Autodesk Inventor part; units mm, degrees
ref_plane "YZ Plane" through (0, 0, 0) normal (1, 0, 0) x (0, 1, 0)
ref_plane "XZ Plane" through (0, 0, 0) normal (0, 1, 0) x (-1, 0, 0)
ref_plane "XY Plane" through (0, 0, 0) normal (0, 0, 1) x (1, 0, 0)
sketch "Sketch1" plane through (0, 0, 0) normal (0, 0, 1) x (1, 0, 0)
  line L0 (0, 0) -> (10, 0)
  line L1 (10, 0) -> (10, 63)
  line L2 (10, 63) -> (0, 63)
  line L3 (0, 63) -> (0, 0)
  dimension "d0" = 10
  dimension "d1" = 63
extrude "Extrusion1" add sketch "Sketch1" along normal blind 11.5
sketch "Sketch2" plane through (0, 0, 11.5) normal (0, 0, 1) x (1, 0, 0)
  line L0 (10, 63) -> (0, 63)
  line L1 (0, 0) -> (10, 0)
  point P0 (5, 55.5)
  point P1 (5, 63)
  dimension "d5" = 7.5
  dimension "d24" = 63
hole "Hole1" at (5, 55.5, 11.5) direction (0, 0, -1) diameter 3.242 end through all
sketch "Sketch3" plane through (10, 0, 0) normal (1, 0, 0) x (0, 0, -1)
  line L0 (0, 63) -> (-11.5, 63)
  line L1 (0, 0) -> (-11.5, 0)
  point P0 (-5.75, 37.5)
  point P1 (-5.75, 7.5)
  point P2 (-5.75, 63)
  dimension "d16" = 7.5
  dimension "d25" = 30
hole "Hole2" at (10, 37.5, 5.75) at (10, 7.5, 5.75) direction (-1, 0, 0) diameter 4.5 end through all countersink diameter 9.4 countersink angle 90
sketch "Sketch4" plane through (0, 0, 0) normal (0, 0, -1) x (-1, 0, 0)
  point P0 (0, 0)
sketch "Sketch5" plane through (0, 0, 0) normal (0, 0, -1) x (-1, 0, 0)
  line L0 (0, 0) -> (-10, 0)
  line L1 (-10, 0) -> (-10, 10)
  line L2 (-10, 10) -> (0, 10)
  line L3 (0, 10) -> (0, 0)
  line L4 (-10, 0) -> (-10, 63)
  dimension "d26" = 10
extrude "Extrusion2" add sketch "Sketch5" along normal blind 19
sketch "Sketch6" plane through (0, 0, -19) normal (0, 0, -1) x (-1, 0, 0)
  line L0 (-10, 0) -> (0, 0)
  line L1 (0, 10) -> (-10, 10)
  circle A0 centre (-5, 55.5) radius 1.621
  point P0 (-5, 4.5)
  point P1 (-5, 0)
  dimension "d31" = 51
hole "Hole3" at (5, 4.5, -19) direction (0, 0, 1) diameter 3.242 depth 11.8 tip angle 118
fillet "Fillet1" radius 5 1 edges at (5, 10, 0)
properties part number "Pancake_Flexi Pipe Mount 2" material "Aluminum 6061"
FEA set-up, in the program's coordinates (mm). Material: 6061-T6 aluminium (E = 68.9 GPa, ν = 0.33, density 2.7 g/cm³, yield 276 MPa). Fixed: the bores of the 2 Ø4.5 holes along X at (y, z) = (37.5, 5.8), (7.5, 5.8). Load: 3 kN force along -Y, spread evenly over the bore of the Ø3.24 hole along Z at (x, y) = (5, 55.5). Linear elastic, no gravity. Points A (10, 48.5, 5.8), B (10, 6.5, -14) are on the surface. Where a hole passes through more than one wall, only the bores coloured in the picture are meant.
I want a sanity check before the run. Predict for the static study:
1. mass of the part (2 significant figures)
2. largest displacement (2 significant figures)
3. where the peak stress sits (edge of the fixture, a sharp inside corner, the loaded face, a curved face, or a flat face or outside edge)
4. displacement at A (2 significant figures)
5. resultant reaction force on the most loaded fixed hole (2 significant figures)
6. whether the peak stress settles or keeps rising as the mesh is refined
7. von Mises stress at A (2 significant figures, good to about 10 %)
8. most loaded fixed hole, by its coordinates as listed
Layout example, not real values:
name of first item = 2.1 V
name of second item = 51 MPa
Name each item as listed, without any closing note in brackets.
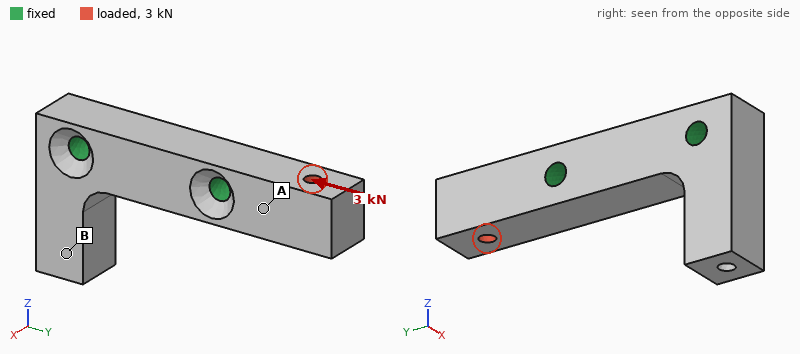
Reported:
mass of the part = 23 g
largest displacement = 10 µm
where the peak stress sits = edge of the fixture
displacement at A = 6.6 µm
resultant reaction force on the most loaded fixed hole = 2.9 kN
whether the peak stress settles or keeps rising as the mesh is refined = keeps rising
von Mises stress at A = 26 MPa
most loaded fixed hole, by its coordinates as listed = (37.5, 5.8)
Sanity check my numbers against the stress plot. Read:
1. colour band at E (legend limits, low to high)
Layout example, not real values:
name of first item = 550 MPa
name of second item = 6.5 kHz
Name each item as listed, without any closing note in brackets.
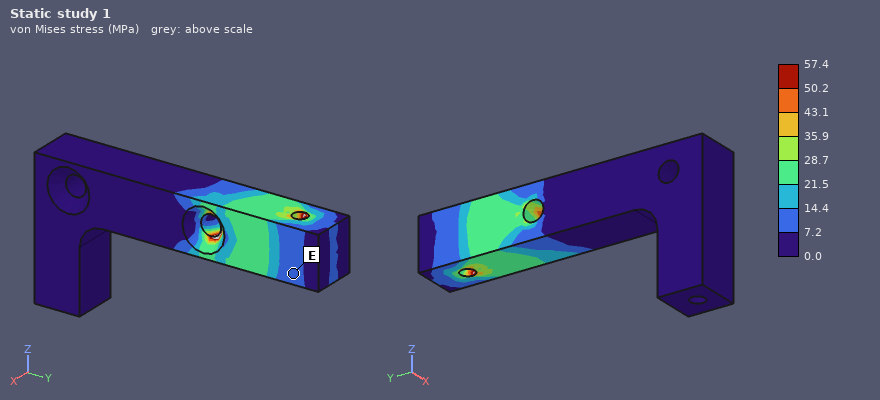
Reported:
colour band at E = 7.2 to 14.4 MPa
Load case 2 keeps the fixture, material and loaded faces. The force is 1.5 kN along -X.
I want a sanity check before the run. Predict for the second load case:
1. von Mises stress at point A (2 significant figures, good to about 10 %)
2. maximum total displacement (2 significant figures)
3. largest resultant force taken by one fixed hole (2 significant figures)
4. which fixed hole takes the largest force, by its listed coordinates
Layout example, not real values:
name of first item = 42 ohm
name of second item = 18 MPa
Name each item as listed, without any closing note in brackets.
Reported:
von Mises stress at point A = 53 MPa
maximum total displacement = 0.10 mm
largest resultant force taken by one fixed hole = 1.7 kN
which fixed hole takes the largest force, by its listed coordinates = (37.5, 5.8)
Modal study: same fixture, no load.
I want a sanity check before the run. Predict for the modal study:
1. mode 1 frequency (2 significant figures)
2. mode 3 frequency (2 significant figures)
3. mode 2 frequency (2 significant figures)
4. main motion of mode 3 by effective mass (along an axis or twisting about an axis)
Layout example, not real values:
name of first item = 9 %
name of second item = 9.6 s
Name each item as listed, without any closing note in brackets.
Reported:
mode 1 frequency = 11 kHz
mode 3 frequency = 12 kHz
mode 2 frequency = 11 kHz
main motion of mode 3 by effective mass = along X
